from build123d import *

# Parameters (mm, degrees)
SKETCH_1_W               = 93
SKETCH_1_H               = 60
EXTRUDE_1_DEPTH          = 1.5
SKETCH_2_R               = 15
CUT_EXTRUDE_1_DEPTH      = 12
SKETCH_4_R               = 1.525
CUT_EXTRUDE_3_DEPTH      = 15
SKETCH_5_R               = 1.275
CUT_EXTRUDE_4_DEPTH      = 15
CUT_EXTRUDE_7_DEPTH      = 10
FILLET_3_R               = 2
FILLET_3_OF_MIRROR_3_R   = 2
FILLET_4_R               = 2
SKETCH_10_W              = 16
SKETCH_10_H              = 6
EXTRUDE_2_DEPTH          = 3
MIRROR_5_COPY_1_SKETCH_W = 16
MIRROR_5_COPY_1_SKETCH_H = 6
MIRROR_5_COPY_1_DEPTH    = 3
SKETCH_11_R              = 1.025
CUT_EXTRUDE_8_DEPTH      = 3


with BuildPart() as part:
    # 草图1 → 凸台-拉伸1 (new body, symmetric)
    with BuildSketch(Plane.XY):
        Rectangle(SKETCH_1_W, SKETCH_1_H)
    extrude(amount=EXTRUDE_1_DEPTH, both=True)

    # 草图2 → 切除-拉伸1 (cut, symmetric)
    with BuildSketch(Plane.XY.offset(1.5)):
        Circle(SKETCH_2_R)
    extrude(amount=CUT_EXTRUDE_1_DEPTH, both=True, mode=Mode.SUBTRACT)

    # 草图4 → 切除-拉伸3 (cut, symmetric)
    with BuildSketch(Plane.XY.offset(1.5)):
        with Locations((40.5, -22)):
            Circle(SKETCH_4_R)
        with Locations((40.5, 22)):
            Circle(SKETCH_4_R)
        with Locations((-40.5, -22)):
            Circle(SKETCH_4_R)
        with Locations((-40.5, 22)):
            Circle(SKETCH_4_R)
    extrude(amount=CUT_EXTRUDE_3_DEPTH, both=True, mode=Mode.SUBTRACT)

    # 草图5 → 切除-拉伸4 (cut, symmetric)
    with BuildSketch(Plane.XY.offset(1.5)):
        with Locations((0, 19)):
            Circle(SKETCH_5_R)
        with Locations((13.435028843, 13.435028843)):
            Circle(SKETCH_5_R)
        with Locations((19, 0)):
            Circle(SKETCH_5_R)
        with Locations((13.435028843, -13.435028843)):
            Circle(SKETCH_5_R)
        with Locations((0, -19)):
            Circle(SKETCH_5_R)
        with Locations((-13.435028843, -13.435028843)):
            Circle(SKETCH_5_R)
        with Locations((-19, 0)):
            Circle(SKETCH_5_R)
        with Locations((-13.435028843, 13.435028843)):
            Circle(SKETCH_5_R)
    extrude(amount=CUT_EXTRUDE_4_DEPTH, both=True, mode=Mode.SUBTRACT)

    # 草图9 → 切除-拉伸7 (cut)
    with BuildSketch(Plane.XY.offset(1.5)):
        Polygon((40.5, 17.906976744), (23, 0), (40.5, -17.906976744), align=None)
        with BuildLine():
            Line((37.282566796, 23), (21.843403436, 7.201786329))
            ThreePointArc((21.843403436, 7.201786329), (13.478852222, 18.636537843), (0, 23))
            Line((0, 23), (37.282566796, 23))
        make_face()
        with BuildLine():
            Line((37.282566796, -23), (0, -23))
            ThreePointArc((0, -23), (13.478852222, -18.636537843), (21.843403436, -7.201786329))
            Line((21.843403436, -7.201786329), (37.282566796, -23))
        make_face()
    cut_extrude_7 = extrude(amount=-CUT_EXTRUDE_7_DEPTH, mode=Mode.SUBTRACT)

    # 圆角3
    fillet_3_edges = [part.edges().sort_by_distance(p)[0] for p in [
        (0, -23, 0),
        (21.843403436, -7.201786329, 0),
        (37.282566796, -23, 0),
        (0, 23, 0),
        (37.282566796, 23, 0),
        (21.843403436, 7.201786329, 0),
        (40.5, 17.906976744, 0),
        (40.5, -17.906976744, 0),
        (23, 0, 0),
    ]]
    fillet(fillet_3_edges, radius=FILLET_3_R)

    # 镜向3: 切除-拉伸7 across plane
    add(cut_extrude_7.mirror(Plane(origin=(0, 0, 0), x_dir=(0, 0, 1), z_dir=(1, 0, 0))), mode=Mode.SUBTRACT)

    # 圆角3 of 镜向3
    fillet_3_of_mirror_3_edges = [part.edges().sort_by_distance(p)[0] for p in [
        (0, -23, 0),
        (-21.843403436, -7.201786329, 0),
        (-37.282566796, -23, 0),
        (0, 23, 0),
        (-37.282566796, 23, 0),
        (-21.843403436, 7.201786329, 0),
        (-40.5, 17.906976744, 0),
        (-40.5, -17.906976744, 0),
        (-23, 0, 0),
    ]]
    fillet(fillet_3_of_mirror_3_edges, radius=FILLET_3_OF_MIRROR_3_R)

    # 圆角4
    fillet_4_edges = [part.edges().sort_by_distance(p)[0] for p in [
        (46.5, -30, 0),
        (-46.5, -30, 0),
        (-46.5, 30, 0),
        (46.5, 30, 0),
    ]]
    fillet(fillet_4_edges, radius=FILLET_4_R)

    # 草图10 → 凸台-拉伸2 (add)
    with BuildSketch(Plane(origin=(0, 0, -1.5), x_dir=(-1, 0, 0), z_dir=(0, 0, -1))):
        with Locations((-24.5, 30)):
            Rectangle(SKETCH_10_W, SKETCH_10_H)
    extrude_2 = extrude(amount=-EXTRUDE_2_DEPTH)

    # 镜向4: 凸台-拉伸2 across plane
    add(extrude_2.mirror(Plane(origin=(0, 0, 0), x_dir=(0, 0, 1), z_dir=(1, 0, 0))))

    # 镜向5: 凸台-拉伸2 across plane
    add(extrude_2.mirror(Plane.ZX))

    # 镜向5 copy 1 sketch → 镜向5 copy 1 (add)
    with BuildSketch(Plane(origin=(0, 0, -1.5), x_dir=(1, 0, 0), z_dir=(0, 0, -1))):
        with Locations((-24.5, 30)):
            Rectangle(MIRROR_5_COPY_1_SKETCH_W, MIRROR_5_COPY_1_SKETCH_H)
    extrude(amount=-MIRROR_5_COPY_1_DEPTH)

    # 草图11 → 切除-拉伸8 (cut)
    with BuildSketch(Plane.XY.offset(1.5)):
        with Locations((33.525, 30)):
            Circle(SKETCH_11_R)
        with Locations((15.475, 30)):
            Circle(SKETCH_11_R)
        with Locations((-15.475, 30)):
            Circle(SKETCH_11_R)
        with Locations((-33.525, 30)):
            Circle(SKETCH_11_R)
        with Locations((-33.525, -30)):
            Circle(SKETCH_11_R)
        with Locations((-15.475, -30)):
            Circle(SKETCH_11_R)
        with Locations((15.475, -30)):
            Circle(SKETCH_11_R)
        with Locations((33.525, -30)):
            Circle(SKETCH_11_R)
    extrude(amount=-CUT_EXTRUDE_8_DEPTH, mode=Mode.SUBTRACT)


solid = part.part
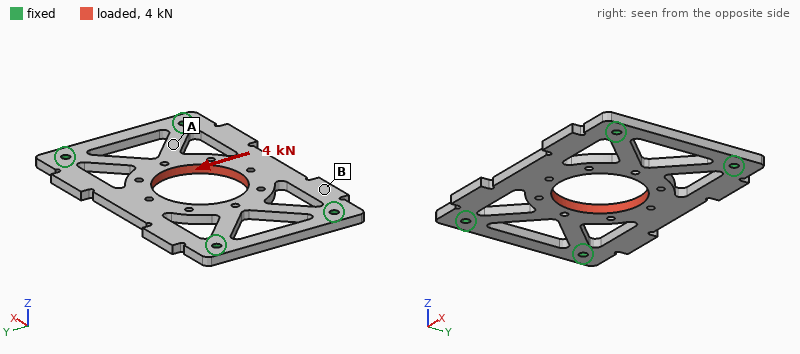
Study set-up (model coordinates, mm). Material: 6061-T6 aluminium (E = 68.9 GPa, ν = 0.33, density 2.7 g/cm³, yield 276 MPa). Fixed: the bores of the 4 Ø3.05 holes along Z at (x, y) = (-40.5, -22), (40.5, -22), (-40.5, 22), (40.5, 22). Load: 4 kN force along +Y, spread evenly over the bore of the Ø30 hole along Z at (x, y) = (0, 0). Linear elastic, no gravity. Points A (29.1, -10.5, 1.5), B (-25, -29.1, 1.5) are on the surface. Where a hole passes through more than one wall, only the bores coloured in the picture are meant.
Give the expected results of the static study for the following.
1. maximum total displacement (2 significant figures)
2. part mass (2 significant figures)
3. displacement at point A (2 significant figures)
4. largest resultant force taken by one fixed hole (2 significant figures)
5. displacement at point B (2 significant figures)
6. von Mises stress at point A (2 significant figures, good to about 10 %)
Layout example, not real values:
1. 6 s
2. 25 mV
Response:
1. 60 µm
2. 29 g
3. 24 µm
4. 1.3 kN
5. 29 µm
6. 69 MPa
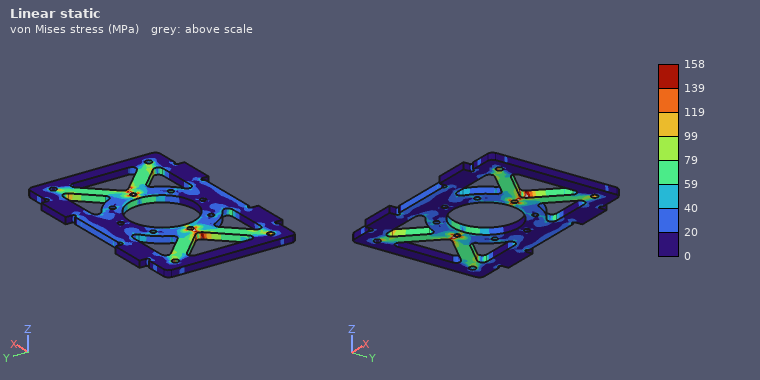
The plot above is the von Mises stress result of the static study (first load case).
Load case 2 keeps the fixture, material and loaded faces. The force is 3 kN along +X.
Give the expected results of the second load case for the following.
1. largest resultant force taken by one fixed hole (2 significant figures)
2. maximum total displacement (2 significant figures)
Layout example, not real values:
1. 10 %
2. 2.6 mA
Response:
1. 810 N
2. 22 µm
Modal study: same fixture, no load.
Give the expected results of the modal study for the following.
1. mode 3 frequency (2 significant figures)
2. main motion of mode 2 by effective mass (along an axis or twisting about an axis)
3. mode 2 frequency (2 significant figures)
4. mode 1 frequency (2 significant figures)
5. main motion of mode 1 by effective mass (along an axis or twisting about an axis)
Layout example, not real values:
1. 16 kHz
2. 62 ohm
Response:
1. 4400 Hz
2. twisting about X
3. 2500 Hz
4. 2000 Hz
5. along Z
